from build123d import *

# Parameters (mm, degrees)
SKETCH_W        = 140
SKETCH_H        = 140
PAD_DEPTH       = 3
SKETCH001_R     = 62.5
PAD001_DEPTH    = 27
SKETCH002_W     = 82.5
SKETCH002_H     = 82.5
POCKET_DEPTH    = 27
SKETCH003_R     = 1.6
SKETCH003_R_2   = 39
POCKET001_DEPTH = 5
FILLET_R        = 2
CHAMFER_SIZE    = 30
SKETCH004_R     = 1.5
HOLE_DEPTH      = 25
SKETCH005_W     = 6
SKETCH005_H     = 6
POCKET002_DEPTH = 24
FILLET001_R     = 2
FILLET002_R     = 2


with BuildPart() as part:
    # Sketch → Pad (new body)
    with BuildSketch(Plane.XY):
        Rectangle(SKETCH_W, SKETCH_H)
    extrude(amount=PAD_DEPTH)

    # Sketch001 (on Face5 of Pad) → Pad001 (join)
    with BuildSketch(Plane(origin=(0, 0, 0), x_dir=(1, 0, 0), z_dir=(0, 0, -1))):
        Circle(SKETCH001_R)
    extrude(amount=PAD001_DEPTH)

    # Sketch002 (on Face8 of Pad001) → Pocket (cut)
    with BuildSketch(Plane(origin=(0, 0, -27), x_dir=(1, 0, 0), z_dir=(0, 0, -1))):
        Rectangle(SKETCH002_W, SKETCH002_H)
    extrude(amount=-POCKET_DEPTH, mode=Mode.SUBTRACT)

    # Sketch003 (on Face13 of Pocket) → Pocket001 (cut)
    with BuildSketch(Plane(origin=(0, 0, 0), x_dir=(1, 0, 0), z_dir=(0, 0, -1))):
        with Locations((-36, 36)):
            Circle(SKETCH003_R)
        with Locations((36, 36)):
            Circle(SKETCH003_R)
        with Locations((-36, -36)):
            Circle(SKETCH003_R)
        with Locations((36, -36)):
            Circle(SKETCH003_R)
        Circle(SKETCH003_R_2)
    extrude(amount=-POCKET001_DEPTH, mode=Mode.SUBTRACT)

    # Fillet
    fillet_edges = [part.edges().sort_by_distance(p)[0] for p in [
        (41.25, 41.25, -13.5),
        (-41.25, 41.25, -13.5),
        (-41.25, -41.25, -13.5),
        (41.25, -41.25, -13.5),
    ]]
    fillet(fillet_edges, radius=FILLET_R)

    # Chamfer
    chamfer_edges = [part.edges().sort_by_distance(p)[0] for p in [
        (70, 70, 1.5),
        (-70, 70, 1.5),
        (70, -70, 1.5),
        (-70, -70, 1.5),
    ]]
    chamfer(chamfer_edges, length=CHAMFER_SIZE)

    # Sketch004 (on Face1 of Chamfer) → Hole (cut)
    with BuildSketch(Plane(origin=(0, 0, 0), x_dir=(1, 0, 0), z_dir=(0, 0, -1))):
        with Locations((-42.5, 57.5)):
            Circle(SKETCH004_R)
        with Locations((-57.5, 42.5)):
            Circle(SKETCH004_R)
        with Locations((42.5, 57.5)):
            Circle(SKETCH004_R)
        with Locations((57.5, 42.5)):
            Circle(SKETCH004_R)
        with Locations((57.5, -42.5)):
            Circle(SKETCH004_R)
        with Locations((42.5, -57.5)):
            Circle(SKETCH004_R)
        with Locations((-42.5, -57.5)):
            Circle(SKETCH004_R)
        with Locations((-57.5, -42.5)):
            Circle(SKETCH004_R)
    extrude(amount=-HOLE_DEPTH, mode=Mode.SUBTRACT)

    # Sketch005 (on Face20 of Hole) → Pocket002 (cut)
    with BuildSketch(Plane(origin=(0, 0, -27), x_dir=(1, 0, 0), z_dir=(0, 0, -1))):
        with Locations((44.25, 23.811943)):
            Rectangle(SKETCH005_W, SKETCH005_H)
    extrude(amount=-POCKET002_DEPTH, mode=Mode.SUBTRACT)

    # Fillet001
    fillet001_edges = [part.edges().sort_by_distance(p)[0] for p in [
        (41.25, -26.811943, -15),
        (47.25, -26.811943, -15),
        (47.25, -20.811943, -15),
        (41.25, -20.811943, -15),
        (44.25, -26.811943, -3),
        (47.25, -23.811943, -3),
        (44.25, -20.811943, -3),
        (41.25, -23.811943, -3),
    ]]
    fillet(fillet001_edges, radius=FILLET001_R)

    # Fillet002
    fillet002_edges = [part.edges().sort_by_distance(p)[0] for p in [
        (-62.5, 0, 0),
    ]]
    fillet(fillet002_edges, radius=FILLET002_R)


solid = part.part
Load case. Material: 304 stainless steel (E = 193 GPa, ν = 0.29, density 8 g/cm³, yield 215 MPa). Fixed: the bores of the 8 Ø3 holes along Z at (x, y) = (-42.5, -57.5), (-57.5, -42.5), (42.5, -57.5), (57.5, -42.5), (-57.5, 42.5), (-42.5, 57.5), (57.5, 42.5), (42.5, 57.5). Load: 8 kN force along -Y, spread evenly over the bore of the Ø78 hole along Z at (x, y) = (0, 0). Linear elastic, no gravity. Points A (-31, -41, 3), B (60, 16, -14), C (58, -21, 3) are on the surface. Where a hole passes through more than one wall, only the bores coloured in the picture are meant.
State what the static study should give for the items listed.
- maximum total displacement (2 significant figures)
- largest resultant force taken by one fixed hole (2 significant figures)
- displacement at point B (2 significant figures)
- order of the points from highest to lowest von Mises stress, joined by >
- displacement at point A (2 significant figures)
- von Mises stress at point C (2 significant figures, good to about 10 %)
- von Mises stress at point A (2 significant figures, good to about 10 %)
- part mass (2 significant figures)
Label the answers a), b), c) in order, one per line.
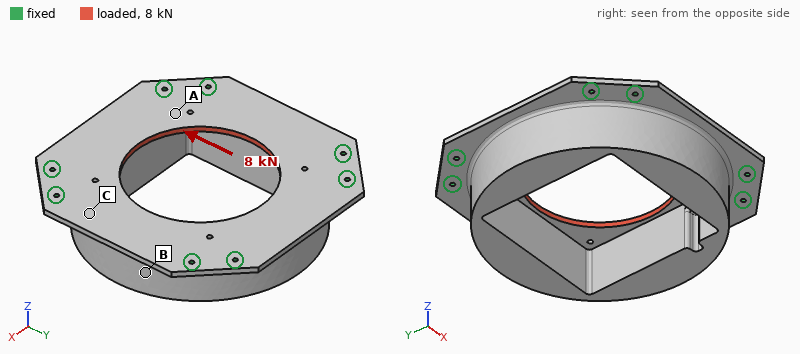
a) 5.8 µm
b) 1.2 kN
c) 1.8 µm
d) A > C > B
e) 3.0 µm
f) 7.7 MPa
g) 14 MPa
h) 1.5 kg
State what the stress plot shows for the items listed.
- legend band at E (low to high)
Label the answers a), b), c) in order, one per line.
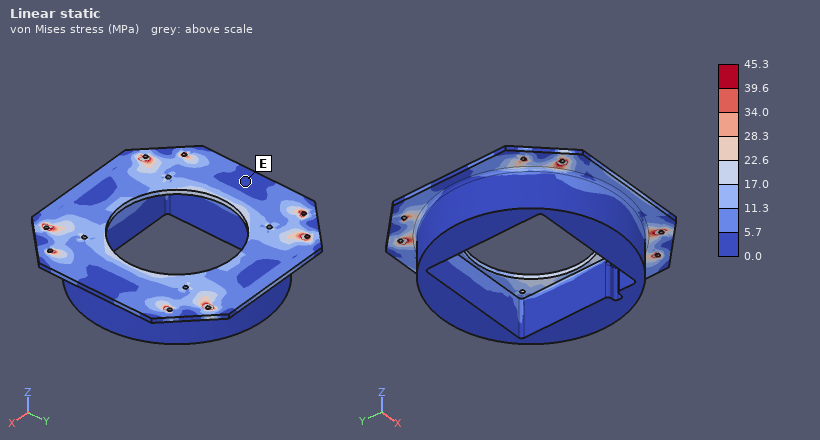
a) 0.0 to 5.7 MPa
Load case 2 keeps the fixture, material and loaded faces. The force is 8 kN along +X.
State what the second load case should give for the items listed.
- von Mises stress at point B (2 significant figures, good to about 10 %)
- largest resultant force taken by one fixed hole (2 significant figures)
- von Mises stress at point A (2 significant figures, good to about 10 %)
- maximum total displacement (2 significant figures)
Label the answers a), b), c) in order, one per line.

a) 4.6 MPa
b) 1.2 kN
c) 11 MPa
d) 5.9 µm
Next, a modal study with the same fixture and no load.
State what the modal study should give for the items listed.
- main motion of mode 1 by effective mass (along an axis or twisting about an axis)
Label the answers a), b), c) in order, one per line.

a) along Z
